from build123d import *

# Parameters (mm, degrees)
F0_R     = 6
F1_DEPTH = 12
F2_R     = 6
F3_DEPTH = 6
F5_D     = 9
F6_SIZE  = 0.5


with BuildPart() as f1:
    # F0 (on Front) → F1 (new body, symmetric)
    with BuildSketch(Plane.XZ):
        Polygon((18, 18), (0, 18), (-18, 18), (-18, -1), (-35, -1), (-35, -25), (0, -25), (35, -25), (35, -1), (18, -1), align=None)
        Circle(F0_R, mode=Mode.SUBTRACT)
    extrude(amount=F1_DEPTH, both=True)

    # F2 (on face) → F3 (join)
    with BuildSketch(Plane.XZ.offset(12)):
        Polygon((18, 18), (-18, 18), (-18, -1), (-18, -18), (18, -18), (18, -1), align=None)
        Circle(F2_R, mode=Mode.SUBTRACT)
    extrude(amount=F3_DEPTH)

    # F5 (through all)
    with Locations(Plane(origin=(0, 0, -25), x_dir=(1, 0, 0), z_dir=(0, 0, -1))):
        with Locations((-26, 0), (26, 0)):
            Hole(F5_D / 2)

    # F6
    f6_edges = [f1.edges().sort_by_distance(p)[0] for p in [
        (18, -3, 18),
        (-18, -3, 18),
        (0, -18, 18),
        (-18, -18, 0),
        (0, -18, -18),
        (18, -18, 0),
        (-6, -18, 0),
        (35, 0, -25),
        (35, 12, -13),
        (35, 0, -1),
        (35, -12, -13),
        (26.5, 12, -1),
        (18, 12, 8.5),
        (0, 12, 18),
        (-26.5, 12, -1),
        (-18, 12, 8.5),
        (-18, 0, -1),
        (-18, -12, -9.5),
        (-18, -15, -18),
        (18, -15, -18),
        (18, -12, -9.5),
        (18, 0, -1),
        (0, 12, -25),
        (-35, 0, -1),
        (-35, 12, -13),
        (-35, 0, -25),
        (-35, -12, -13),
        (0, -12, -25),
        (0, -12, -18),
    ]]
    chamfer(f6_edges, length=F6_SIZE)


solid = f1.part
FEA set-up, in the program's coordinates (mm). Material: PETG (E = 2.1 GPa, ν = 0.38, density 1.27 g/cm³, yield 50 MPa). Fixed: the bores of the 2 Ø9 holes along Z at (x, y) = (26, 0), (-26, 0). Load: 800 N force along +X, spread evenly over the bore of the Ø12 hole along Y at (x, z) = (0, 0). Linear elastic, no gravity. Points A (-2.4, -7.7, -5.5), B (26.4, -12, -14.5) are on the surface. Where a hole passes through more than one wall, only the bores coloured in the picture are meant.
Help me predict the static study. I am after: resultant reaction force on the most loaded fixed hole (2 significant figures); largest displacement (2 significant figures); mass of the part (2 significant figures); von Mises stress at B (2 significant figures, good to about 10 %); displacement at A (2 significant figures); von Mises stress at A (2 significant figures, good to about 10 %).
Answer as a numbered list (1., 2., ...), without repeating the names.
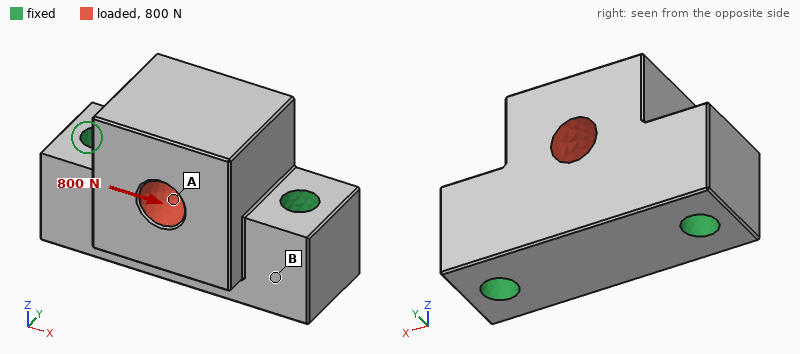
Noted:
1. 440 N
2. 20 µm
3. 74 g
4. 0.41 MPa
5. 9.5 µm
6. 1.4 MPa
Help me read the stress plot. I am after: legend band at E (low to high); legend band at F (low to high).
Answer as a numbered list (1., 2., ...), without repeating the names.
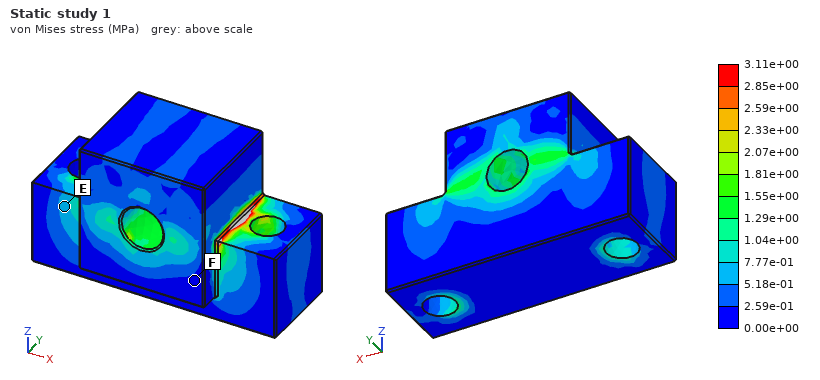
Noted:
1. 5.18e-01 to 7.77e-01 MPa
2. 0.00e+00 to 2.59e-01 MPa
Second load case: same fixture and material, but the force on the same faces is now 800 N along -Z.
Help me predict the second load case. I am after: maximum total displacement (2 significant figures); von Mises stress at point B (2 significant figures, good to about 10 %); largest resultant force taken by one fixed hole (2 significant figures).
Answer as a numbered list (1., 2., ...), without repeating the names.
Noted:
1. 29 µm
2. 0.50 MPa
3. 410 N
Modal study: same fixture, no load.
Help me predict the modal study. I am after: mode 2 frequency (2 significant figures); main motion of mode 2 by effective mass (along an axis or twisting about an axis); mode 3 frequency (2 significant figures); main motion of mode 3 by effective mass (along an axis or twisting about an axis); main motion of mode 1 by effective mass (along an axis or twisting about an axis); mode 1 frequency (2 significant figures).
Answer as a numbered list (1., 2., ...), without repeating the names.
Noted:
1. 4900 Hz
2. along X
3. 5100 Hz
4. along Z
5. along Y
6. 2600 Hz
